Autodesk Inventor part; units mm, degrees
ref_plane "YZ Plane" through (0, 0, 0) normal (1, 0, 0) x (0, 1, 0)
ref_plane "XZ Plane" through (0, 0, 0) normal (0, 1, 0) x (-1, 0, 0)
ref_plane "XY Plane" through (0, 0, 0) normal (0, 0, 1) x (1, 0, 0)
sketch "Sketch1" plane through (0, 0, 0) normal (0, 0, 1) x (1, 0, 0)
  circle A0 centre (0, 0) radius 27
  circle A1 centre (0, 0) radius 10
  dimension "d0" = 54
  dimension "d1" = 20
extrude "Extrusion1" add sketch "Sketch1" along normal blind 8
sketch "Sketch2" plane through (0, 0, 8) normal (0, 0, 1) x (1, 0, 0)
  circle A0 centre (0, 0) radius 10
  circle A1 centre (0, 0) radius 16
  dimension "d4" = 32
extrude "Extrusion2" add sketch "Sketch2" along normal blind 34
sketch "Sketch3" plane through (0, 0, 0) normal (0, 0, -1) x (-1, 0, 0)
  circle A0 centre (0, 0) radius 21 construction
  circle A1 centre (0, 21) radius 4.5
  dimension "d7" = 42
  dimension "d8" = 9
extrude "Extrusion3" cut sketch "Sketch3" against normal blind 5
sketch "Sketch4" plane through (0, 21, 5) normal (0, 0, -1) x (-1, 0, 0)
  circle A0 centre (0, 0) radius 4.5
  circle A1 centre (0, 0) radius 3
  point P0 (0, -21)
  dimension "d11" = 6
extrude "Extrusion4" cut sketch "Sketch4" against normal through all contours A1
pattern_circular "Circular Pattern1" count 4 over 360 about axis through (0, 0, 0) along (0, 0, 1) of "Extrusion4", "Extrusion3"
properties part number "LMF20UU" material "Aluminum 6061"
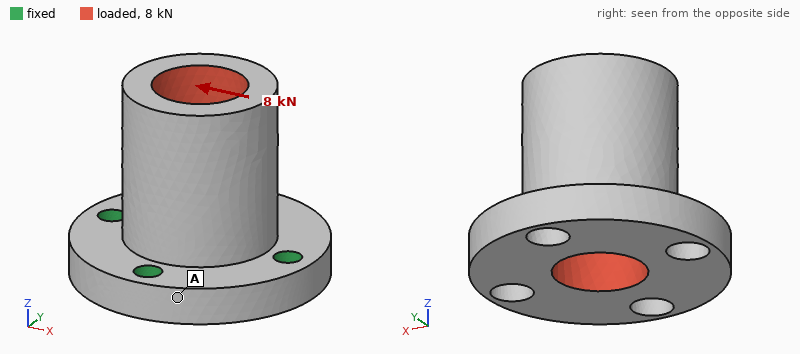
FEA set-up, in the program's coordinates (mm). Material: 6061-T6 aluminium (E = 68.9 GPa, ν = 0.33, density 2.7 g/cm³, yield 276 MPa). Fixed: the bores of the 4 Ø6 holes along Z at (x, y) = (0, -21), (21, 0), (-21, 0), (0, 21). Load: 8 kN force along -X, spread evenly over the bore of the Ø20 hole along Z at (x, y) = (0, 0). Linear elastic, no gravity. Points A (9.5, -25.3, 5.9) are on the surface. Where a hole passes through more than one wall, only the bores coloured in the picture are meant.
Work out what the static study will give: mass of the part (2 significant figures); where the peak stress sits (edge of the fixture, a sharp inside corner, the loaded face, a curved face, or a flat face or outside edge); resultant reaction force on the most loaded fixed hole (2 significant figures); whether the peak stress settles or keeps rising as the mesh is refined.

83 g
edge of the fixture
3.4 kN
keeps rising
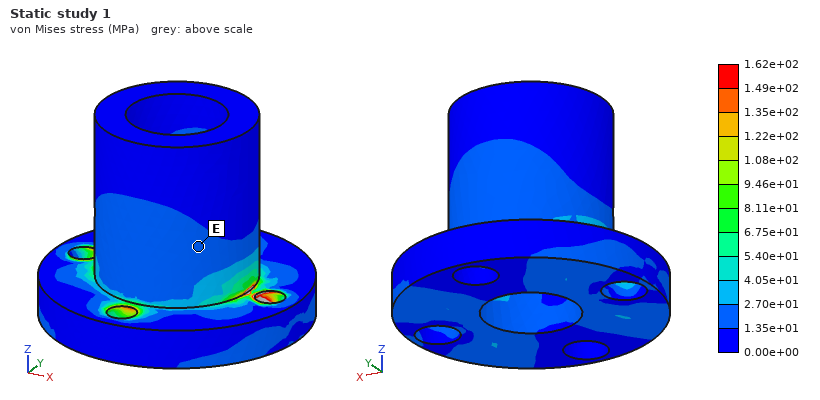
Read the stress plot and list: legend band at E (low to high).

1.35e+01 to 2.70e+01 MPa
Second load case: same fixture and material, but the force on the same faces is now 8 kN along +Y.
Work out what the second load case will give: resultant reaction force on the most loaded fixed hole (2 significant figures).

3.4 kN
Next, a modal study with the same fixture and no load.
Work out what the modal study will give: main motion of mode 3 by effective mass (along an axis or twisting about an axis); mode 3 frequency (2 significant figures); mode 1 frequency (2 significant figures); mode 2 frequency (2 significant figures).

along Z
16 kHz
8900 Hz
8900 Hz
